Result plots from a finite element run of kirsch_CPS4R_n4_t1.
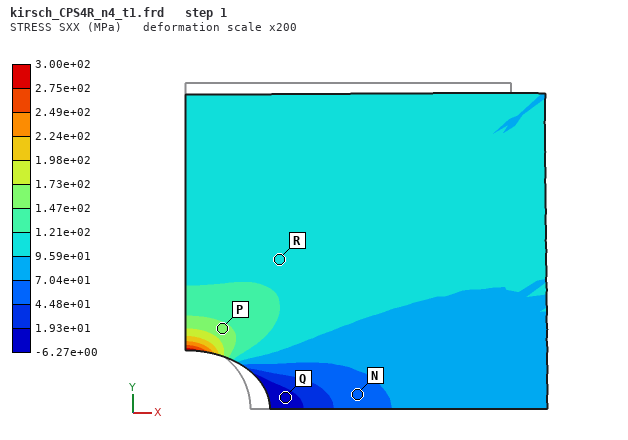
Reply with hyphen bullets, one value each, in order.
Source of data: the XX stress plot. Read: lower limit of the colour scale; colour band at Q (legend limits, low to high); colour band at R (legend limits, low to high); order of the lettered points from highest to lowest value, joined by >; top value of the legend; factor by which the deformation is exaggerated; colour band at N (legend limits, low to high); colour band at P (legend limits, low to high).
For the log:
- -6.27e+00 MPa
- -6.27e+00 to 1.93e+01 MPa
- 9.59e+01 to 1.21e+02 MPa
- P > R > N > Q
- 3.00e+02 MPa
- 200
- 4.48e+01 to 7.04e+01 MPa
- 1.47e+02 to 1.73e+02 MPa
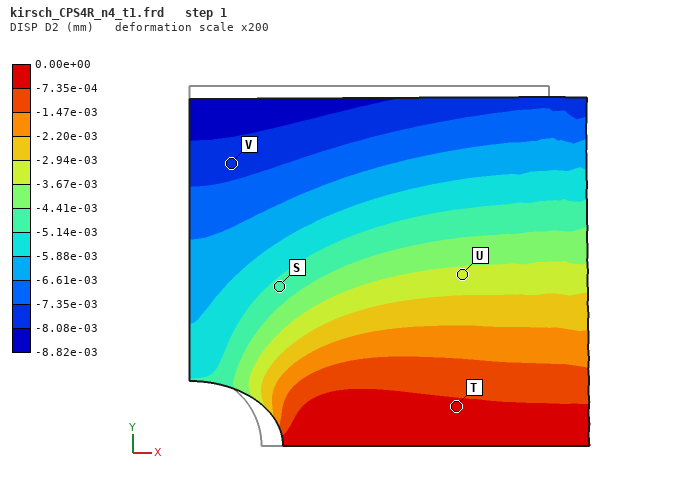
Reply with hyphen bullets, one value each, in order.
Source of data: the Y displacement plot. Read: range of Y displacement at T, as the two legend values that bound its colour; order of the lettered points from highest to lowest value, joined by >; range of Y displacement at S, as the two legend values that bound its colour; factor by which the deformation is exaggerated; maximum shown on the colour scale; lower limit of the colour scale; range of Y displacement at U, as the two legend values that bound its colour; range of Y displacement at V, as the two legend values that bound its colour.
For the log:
- -7.35e-04 to 0.00e+00 mm
- T > U > S > V
- -5.14e-03 to -4.41e-03 mm
- 200
- 0.00e+00 mm
- -8.82e-03 mm
- -3.67e-03 to -2.94e-03 mm
- -8.08e-03 to -7.35e-03 mm
